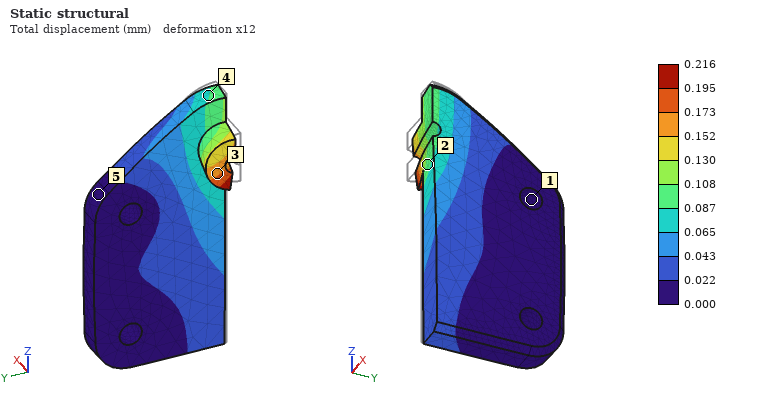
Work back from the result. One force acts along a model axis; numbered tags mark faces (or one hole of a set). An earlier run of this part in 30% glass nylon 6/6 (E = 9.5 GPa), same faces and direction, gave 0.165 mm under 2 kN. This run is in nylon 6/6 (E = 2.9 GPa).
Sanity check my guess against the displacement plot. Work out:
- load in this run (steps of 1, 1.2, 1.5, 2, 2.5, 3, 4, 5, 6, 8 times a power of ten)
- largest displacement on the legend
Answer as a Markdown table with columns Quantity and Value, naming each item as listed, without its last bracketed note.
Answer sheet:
| Quantity | Value |
|---|---|
| load in this run | 800 N |
| largest displacement on the legend | 0.216 mm |
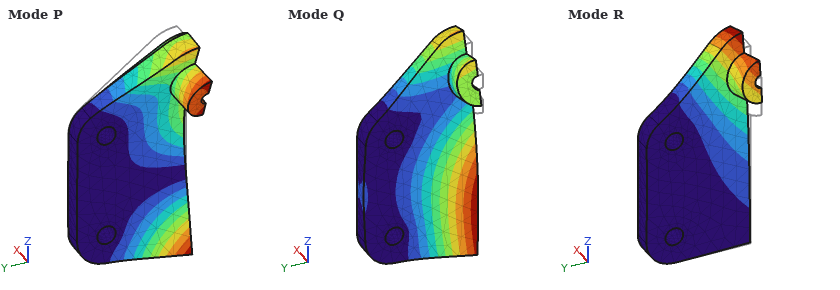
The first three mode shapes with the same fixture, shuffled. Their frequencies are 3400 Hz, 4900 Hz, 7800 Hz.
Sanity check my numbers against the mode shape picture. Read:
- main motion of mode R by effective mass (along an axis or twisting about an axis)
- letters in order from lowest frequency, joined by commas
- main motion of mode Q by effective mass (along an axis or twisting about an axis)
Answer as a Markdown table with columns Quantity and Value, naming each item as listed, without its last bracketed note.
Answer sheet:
| Quantity | Value |
|---|---|
| main motion of mode R by effective mass | along X |
| letters in order from lowest frequency, joined by commas | R, Q, P |
| main motion of mode Q by effective mass | along X |
